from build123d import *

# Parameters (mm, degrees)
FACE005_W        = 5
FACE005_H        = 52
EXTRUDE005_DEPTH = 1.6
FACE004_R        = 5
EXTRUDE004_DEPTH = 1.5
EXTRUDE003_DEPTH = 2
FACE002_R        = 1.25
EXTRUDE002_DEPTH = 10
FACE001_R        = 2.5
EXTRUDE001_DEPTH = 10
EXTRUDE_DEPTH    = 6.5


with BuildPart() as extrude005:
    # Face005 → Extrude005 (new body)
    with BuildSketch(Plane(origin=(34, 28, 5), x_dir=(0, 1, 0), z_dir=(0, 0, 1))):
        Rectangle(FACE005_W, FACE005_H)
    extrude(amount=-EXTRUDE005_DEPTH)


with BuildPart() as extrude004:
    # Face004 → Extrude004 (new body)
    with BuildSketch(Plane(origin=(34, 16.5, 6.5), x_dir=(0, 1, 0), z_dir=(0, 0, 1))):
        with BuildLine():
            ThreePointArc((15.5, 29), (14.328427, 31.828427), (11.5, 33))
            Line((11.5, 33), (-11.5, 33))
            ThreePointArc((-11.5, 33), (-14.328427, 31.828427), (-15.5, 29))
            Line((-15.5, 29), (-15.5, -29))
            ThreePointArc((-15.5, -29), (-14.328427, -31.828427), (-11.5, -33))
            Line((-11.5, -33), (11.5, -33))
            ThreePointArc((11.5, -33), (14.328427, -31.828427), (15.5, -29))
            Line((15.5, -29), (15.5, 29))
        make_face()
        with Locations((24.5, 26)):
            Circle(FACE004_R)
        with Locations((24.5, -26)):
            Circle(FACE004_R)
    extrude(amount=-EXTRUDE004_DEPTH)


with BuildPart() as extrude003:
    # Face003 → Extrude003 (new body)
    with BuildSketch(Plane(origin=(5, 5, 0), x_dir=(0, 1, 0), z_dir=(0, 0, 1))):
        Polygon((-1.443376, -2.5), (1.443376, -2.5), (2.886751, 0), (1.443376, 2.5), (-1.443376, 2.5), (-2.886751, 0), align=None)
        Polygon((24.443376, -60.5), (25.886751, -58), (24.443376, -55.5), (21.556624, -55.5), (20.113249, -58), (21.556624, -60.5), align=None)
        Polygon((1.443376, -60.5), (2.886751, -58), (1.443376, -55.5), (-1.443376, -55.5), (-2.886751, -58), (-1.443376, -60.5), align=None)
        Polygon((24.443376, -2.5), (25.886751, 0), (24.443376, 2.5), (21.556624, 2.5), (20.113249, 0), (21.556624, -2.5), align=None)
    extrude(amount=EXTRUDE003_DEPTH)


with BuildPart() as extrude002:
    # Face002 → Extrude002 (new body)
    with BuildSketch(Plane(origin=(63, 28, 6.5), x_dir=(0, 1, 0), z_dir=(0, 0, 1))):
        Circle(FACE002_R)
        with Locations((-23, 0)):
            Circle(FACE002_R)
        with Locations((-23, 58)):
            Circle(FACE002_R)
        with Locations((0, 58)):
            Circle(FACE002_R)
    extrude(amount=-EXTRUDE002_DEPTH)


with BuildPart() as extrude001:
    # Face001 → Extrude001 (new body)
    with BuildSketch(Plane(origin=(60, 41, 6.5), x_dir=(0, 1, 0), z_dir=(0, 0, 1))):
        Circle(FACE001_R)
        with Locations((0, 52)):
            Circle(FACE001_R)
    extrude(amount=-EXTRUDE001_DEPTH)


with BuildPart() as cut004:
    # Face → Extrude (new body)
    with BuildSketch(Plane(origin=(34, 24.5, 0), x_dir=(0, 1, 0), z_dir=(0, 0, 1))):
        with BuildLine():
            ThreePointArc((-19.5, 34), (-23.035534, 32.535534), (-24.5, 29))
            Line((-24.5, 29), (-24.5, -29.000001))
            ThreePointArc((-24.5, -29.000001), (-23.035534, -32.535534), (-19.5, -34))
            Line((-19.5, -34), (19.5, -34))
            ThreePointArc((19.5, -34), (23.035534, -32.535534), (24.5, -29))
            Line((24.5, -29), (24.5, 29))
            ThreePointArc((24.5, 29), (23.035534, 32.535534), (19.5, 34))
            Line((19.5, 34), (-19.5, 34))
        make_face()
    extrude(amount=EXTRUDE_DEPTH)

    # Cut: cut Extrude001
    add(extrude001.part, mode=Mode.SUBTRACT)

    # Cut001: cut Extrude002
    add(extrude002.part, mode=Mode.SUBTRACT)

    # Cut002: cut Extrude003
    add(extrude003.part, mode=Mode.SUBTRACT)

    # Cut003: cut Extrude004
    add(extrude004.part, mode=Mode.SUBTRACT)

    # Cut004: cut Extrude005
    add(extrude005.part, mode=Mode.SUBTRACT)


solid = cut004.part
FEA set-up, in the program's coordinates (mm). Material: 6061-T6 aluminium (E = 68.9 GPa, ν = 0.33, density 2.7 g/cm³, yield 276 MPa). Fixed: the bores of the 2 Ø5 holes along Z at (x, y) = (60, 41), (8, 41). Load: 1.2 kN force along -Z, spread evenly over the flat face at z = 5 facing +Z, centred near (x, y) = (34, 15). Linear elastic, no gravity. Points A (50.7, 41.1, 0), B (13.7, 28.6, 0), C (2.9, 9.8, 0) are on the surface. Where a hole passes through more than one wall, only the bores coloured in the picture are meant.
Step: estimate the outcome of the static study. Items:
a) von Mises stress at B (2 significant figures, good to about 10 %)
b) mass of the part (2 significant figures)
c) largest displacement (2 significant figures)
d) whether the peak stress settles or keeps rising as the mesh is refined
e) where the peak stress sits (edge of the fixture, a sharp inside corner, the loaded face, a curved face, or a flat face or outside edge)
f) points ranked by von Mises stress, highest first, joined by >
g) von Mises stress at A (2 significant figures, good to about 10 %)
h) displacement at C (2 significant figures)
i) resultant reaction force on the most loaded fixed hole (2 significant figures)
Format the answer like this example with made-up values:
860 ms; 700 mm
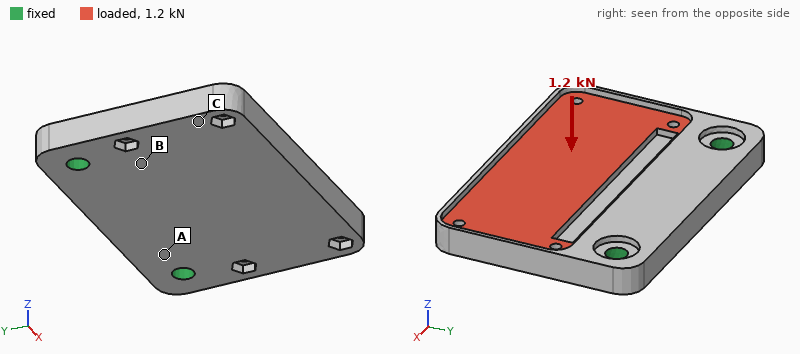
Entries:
95 MPa; 47 g; 0.41 mm; keeps rising; edge of the fixture; B > A > C; 52 MPa; 0.24 mm; 610 N
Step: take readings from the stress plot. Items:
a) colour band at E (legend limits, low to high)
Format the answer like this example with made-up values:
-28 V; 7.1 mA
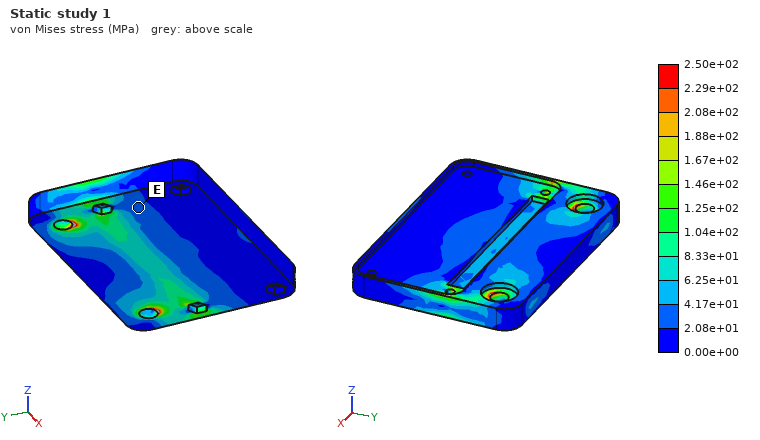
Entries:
2.08e+01 to 4.17e+01 MPa
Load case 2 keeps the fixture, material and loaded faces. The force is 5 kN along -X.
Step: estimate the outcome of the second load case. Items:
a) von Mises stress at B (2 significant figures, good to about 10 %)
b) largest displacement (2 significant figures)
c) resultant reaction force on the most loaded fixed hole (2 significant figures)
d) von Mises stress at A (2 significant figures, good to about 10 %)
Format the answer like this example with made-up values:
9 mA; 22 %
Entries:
38 MPa; 94 µm; 3.5 kN; 23 MPa
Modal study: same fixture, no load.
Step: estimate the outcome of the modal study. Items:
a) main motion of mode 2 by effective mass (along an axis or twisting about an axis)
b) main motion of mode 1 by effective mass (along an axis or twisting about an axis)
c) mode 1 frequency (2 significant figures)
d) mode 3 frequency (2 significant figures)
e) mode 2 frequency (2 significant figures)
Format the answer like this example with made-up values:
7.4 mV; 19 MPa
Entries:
twisting about Y; along Z; 2100 Hz; 8100 Hz; 4200 Hz
